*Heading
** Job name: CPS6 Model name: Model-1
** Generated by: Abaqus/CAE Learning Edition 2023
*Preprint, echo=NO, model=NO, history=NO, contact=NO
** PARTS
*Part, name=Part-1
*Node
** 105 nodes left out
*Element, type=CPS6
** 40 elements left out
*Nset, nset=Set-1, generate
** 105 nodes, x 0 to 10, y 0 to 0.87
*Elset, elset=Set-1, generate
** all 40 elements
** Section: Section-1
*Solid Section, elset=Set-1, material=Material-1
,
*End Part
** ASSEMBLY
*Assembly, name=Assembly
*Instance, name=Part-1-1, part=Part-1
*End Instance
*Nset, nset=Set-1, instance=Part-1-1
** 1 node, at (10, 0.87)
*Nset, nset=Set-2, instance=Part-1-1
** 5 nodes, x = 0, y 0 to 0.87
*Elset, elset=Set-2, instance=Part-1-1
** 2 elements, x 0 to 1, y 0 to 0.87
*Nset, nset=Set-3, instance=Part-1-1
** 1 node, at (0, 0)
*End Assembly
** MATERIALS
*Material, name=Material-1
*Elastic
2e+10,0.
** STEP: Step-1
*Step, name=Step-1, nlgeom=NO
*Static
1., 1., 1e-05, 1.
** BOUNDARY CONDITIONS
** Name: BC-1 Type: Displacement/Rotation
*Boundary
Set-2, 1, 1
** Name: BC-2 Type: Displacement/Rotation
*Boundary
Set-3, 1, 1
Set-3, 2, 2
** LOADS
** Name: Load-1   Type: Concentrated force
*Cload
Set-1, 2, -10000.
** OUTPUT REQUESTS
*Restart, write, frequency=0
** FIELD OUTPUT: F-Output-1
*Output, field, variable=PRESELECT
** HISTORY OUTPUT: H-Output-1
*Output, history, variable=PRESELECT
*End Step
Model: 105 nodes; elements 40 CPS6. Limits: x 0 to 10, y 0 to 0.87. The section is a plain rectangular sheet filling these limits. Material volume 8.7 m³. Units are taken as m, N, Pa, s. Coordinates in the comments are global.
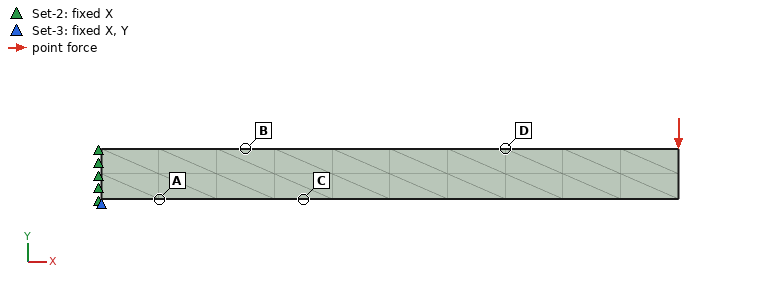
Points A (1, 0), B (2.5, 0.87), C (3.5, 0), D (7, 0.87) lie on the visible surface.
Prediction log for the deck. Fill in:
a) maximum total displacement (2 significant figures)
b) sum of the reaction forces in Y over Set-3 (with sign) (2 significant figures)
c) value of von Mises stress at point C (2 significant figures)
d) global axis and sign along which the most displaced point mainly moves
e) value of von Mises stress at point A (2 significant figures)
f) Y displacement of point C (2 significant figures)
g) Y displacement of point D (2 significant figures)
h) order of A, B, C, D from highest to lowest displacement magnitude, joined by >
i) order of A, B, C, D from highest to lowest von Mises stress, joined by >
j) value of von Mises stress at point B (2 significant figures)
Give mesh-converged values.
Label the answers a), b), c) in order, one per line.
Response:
a) 0.0031 m
b) 10000 N
c) 5.2e+05 Pa
d) -Y
e) 7.1e+05 Pa
f) -5.0e-04 m
g) -0.0017 m
h) D > C > B > A
i) A > B > C > D
j) 5.9e+05 Pa
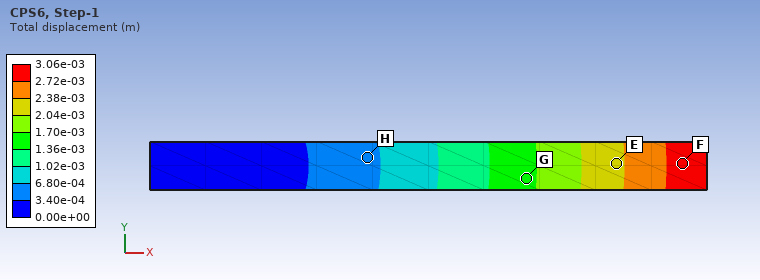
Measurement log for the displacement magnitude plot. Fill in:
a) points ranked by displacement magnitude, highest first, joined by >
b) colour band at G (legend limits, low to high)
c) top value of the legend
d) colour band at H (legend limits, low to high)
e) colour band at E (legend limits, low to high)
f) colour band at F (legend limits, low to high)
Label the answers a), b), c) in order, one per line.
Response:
a) F > E > G > H
b) 1.36e-03 to 1.70e-03 m
c) 3.06e-03 m
d) 3.40e-04 to 6.80e-04 m
e) 2.04e-03 to 2.38e-03 m
f) 2.72e-03 to 3.06e-03 m
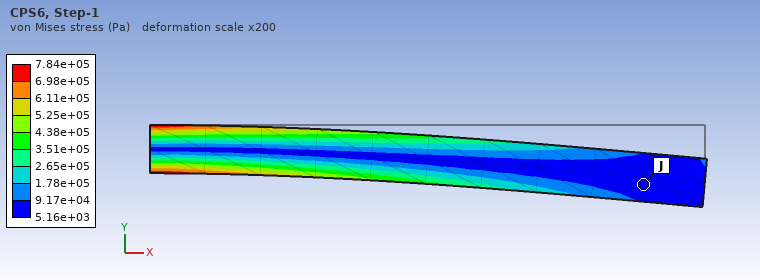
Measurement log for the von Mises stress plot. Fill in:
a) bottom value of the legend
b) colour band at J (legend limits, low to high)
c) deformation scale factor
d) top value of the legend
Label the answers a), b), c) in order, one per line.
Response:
a) 5.16e+03 Pa
b) 5.16e+03 to 9.17e+04 Pa
c) 200
d) 7.84e+05 Pa
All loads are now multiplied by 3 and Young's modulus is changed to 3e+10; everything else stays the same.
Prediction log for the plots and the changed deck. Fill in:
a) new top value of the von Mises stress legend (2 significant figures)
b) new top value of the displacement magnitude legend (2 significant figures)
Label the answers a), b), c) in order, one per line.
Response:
a) 2.4e+06 Pa
b) 0.0061 m
